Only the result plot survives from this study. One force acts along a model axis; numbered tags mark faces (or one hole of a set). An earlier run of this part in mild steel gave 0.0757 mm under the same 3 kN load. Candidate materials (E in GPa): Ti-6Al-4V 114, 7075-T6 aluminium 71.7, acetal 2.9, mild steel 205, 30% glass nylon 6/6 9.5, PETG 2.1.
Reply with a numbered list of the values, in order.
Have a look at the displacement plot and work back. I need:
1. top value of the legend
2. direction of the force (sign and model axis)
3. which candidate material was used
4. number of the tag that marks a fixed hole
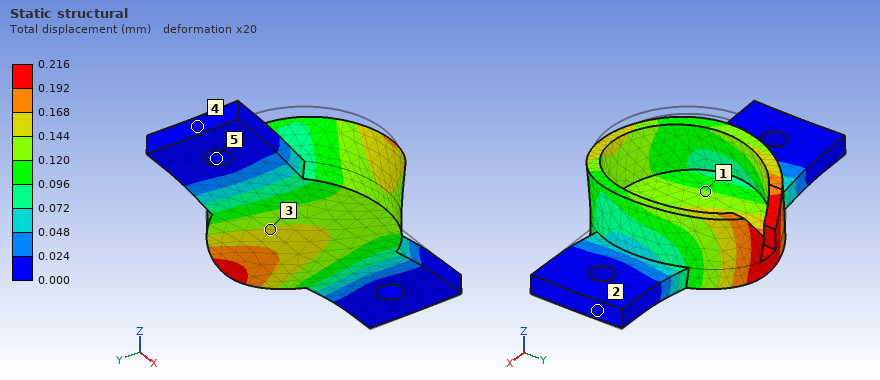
1. 0.216 mm
2. -Z
3. 7075-T6 aluminium
4. 5
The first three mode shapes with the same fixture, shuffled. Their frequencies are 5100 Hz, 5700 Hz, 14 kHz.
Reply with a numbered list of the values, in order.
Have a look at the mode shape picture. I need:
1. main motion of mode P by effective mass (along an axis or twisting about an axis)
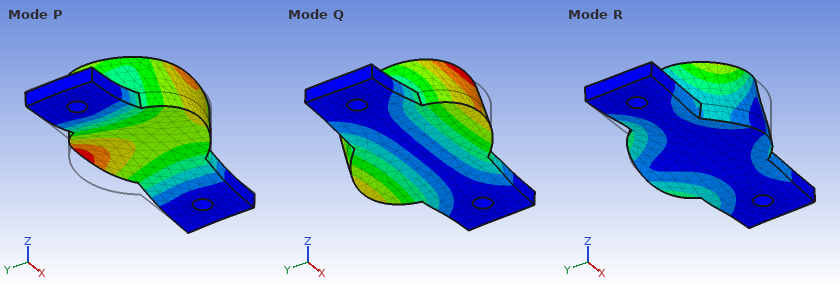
1. along Z
